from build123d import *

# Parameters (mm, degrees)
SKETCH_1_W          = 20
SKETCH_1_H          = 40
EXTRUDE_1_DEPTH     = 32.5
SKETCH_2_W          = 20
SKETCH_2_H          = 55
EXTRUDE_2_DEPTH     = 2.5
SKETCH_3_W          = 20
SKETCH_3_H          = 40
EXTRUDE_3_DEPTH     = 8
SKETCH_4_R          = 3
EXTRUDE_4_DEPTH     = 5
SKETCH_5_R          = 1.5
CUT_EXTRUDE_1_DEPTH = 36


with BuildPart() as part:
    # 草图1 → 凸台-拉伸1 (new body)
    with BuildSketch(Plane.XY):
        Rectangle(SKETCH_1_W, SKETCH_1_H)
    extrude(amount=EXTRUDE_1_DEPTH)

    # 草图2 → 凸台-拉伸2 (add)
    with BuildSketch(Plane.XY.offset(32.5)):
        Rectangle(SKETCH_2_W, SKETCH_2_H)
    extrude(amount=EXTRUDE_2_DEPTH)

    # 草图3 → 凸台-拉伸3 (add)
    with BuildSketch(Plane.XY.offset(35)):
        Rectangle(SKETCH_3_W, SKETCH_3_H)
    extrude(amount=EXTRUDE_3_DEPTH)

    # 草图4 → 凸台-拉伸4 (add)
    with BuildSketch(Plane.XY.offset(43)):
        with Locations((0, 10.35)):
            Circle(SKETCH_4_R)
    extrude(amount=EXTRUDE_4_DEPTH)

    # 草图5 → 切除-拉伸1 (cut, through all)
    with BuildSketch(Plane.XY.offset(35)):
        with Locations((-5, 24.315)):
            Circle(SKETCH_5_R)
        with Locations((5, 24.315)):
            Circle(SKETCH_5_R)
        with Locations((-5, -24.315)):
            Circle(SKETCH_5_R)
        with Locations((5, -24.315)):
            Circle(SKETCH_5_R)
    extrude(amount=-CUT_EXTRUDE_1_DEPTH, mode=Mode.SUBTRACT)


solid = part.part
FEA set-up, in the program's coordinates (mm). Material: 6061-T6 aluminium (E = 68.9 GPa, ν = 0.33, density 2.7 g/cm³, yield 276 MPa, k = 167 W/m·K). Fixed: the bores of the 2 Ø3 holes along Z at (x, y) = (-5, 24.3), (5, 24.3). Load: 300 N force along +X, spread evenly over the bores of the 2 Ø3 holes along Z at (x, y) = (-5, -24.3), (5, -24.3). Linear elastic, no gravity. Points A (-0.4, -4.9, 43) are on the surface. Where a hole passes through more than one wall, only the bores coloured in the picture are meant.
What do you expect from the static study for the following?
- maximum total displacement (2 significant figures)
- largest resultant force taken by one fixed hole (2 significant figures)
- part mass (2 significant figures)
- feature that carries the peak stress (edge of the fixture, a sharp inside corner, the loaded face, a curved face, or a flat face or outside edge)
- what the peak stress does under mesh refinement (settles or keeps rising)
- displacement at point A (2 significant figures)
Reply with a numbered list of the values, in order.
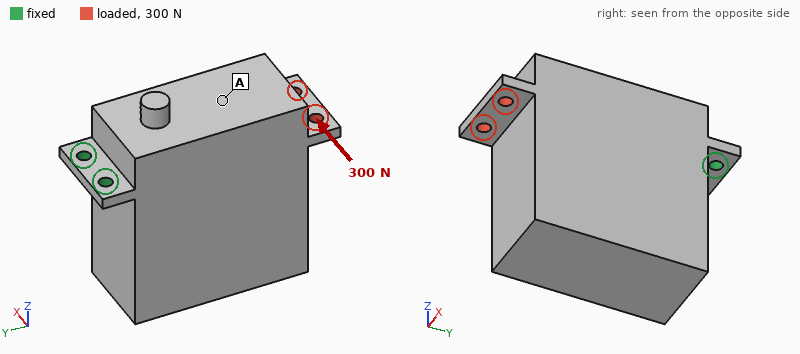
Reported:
1. 67 µm
2. 1.2 kN
3. 95 g
4. edge of the fixture
5. keeps rising
6. 33 µm
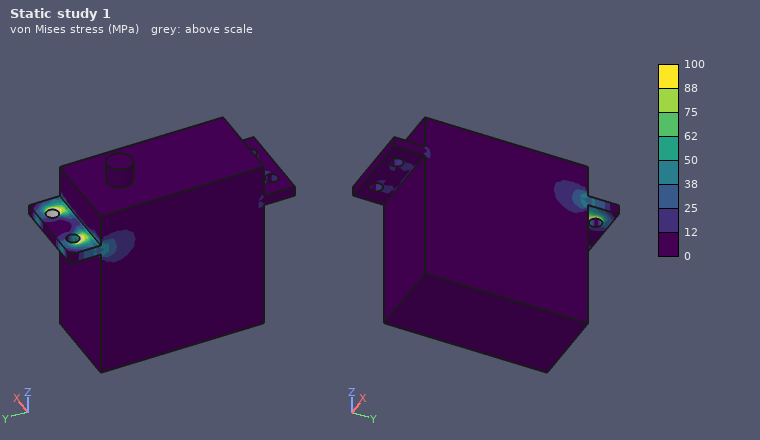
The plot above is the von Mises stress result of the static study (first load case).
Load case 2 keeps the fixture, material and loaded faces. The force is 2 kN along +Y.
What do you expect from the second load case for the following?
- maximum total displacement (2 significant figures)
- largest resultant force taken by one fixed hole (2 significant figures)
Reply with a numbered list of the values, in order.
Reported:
1. 16 µm
2. 1.0 kN
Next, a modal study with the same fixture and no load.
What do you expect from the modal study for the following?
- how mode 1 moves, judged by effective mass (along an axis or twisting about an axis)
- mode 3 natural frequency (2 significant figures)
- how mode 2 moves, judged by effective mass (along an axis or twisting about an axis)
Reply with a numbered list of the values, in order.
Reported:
1. along Z
2. 2900 Hz
3. along X
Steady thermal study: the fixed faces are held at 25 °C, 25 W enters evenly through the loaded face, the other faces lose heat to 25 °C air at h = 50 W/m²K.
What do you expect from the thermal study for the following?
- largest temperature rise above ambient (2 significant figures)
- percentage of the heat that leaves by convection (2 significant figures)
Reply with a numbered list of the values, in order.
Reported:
1. 45 K
2. 26 %
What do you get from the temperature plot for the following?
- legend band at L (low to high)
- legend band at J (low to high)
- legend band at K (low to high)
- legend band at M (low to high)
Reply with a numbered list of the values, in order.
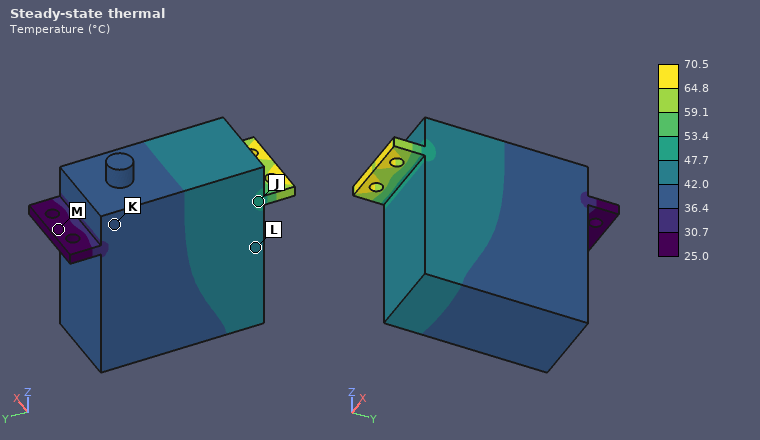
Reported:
1. 42.0 to 47.7 °C
2. 47.7 to 53.4 °C
3. 36.4 to 42.0 °C
4. 25.0 to 30.7 °C
